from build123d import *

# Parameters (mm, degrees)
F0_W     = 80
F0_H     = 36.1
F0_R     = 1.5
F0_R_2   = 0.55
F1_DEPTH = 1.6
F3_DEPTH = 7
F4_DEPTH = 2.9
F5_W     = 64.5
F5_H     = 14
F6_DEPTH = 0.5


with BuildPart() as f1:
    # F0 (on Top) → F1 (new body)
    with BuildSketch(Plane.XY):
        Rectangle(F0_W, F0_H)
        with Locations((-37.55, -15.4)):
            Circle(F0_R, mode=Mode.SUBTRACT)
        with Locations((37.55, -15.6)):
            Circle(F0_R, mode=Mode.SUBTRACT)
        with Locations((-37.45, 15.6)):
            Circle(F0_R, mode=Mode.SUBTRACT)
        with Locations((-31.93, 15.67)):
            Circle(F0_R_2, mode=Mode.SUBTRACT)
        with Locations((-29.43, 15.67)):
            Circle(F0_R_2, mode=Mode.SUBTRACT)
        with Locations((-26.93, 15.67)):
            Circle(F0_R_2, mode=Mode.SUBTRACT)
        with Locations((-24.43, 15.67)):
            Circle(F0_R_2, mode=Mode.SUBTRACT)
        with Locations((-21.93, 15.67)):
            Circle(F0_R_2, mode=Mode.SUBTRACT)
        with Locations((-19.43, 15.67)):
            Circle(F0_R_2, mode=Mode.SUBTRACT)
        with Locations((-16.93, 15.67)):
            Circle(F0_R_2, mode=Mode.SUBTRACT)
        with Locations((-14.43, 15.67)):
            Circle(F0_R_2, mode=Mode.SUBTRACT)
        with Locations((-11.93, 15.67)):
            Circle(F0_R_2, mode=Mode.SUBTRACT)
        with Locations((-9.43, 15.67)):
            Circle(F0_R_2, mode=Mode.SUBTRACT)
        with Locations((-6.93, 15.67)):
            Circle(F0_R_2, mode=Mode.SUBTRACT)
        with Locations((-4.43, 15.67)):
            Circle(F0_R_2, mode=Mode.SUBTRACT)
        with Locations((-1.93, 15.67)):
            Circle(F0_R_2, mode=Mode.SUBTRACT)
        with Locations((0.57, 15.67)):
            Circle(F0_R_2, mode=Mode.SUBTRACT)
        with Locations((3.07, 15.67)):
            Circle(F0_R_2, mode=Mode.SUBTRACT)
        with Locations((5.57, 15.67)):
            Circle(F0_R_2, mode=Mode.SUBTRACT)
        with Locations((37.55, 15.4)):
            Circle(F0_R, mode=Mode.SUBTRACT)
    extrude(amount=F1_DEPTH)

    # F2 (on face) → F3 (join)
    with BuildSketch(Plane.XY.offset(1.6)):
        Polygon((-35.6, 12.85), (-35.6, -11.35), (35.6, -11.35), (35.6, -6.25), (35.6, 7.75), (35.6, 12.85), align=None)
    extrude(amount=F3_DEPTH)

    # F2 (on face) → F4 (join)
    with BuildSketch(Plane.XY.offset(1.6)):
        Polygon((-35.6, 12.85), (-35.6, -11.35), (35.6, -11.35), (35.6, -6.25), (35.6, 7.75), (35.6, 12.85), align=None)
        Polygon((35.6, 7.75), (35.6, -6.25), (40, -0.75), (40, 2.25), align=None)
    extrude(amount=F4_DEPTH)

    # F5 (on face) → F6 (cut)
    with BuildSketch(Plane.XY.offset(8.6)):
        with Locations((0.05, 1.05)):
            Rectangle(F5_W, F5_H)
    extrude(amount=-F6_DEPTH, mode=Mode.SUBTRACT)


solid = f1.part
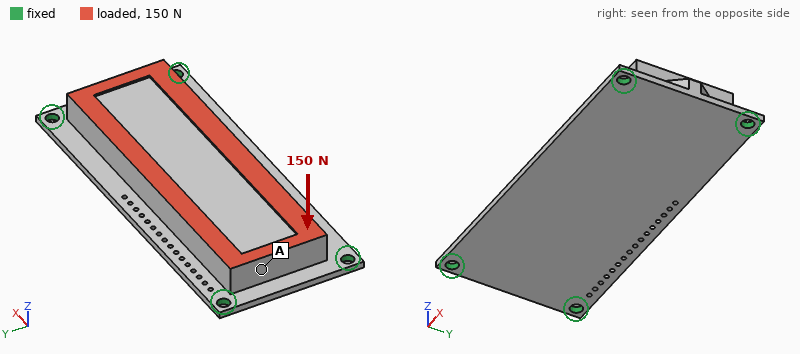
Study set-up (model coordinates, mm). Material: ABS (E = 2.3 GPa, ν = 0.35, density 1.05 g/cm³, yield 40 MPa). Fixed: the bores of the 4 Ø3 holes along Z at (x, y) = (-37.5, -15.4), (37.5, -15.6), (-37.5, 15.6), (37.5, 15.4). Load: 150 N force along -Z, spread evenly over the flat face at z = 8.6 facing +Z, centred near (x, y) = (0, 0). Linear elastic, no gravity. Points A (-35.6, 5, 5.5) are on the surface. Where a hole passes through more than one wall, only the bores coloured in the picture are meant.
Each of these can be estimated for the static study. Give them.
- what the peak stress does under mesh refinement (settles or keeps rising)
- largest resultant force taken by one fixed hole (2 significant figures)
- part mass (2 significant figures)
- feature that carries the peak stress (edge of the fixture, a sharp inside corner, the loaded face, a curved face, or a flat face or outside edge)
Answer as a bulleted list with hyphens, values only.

- keeps rising
- 70 N
- 17 g
- edge of the fixture
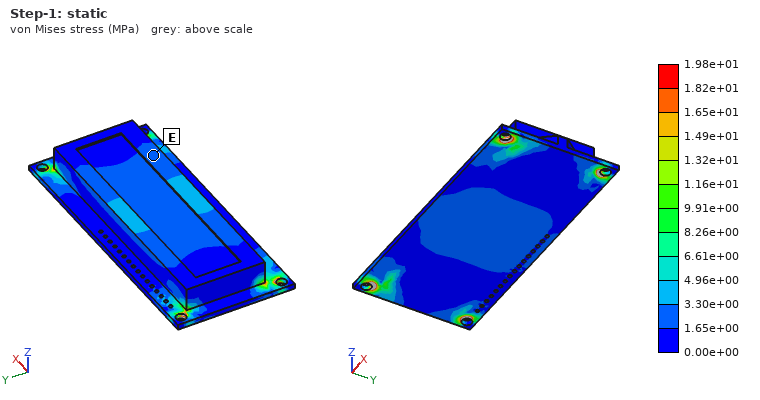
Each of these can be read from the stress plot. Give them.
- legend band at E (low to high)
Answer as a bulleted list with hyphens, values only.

- 1.65e+00 to 3.30e+00 MPa
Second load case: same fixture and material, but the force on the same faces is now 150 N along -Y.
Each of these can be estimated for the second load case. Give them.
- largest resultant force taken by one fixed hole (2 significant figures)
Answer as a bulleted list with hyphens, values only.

- 52 N
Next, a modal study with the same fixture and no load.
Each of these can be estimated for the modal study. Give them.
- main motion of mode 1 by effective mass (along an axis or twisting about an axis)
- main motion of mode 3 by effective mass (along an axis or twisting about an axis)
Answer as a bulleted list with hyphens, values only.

- along Z
- twisting about Y
